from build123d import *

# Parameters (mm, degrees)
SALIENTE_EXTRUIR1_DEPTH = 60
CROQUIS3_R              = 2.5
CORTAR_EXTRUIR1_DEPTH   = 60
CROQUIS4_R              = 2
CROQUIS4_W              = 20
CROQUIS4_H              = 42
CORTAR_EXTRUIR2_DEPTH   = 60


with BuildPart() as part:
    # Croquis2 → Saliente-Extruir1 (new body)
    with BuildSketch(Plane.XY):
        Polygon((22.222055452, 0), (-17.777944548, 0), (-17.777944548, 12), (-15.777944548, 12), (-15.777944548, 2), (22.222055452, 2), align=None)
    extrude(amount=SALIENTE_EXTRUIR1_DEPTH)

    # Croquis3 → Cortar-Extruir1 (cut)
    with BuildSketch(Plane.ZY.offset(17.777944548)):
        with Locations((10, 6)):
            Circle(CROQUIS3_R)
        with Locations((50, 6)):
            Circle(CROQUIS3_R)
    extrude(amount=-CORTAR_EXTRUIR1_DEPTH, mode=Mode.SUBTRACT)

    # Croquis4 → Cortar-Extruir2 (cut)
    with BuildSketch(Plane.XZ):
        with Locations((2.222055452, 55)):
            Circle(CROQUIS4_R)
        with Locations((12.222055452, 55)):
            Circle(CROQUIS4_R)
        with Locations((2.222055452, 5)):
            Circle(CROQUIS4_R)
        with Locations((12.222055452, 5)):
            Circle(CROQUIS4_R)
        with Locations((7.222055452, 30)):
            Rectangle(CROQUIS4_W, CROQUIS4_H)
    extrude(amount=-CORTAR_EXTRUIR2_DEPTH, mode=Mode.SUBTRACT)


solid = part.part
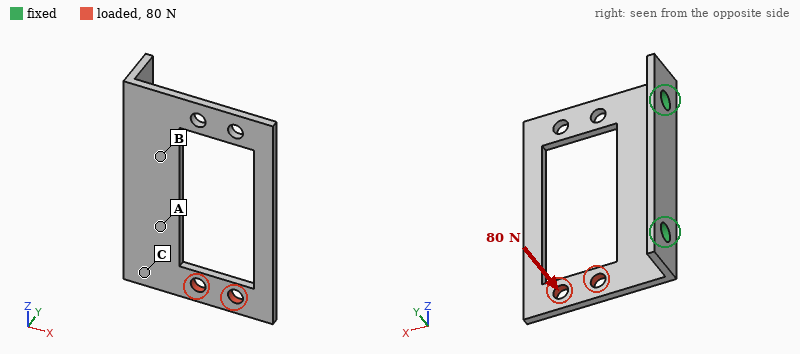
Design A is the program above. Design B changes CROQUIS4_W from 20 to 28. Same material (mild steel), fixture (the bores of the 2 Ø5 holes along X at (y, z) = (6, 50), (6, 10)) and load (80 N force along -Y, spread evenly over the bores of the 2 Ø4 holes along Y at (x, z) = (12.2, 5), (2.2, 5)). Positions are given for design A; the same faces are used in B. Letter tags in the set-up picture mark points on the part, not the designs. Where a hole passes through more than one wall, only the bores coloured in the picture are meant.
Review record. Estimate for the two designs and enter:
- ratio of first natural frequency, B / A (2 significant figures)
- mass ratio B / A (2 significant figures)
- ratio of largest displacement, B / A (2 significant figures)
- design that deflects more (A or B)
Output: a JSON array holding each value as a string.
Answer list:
["1.2", "0.84", "1.4", "B"]
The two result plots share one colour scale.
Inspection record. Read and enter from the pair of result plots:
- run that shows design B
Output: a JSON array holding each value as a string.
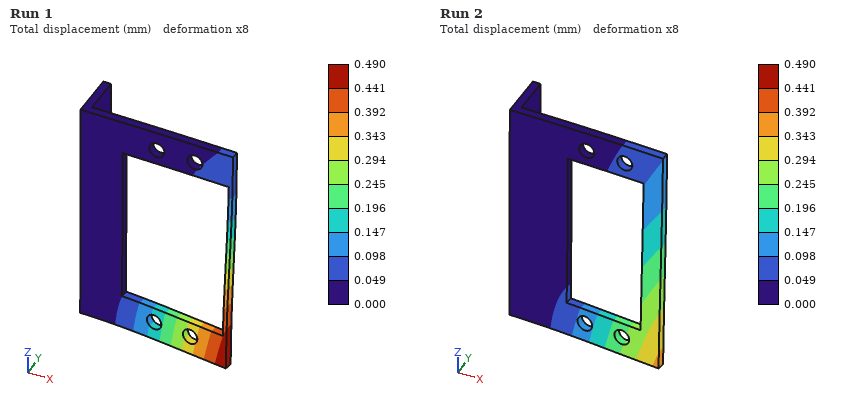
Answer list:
["Run 1"]
